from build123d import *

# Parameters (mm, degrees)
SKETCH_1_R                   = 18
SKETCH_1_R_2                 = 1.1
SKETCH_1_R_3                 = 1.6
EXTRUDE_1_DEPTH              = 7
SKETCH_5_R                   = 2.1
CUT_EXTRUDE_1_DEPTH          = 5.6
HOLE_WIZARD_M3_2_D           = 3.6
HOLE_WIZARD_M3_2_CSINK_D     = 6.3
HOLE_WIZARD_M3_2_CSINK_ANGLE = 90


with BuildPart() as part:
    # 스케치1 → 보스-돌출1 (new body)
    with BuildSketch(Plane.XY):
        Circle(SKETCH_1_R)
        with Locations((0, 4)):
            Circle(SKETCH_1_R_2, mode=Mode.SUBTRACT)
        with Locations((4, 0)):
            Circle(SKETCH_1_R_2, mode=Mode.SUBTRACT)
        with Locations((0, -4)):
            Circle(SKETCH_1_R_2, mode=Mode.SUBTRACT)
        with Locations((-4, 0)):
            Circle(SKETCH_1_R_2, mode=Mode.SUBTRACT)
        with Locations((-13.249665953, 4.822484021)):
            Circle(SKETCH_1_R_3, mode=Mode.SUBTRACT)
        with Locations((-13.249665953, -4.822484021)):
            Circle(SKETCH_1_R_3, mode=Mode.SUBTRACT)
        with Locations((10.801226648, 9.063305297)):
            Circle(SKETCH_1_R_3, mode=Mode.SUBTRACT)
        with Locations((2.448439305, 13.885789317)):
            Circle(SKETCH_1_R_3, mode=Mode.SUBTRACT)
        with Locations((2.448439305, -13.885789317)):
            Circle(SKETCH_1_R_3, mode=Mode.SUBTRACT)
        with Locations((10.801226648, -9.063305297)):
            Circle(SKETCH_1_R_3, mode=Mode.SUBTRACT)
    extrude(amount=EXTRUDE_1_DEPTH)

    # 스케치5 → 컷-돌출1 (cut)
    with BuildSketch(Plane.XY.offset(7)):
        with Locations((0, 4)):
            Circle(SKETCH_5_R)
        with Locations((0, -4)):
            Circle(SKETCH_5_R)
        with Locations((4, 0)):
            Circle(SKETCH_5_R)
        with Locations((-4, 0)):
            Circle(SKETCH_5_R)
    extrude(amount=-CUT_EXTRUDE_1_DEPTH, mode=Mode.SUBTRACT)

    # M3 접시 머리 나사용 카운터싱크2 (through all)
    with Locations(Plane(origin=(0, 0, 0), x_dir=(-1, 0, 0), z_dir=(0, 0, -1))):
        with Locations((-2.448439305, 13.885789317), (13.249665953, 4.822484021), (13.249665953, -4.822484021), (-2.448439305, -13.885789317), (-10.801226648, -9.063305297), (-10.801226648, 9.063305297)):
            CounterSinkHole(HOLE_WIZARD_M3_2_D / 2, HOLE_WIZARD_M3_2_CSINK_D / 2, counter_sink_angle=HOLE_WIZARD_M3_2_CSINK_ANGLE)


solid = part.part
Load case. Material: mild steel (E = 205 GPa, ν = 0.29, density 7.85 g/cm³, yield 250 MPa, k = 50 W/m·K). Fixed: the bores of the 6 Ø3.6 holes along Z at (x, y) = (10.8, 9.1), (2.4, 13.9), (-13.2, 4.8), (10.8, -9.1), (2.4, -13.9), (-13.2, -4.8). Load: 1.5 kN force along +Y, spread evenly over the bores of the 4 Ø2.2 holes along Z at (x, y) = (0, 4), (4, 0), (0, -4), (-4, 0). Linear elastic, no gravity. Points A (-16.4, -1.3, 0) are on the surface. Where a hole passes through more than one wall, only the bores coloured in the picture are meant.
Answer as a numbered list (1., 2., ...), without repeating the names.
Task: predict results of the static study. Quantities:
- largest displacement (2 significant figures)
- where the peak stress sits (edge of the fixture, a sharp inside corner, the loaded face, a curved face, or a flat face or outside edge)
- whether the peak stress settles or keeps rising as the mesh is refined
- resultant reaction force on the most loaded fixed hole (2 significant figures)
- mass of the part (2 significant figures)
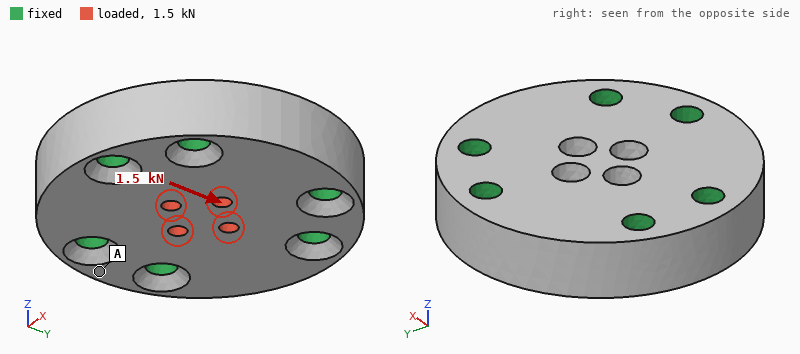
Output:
1. 1.2 µm
2. a sharp inside corner
3. keeps rising
4. 400 N
5. 49 g
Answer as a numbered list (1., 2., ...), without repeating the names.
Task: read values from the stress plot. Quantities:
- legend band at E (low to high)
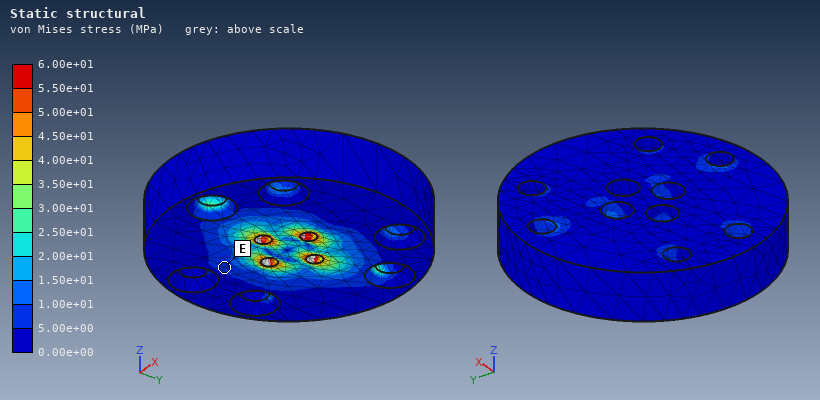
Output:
1. 5.00e+00 to 1.00e+01 MPa
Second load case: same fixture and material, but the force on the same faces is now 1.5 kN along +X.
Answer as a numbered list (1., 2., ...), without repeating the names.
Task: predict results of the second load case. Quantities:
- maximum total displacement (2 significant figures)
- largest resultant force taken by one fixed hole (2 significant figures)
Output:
1. 1.2 µm
2. 360 N
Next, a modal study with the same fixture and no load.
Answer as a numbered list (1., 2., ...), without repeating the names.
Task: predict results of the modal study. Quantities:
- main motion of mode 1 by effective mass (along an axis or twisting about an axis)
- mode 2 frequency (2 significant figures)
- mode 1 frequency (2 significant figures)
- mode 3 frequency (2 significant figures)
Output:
1. along Z
2. 57 kHz
3. 54 kHz
4. 57 kHz
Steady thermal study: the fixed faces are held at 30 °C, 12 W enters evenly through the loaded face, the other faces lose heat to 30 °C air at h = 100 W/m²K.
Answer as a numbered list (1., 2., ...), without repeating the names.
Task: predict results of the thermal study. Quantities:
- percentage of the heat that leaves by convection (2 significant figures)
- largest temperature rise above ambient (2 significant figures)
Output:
1. 5.7 %
2. 18 K
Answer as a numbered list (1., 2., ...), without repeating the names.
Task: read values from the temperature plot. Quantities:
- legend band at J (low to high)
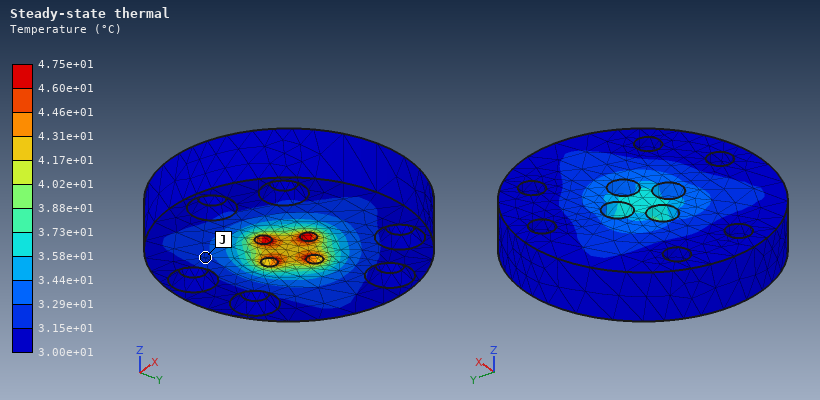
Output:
1. 3.15e+01 to 3.29e+01 °C
